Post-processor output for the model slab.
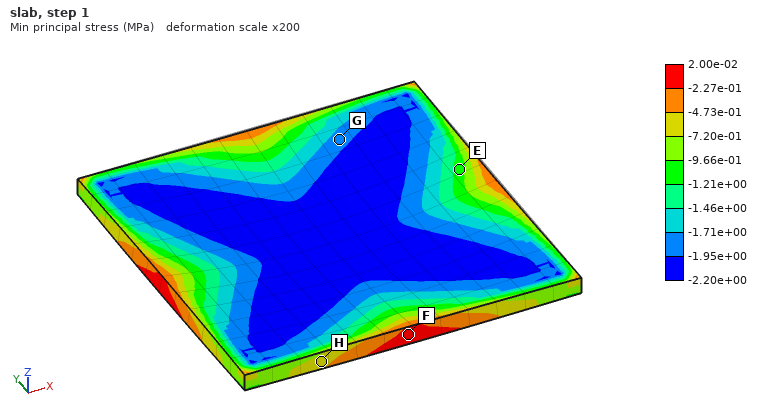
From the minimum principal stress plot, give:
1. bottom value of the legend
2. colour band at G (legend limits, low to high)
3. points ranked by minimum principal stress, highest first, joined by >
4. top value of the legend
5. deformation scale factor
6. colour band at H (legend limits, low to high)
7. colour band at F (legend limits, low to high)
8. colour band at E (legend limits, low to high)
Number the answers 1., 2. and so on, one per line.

1. -2.20e+00 MPa
2. -1.95e+00 to -1.71e+00 MPa
3. F > H > E > G
4. 2.00e-02 MPa
5. 200
6. -7.20e-01 to -4.73e-01 MPa
7. -2.27e-01 to 2.00e-02 MPa
8. -1.21e+00 to -9.66e-01 MPa
